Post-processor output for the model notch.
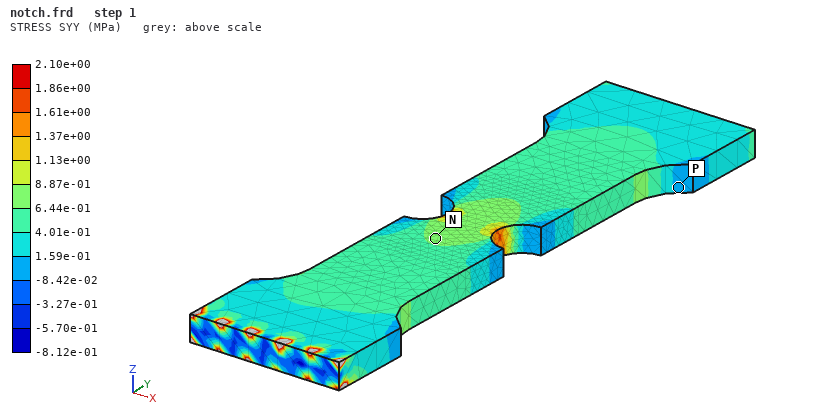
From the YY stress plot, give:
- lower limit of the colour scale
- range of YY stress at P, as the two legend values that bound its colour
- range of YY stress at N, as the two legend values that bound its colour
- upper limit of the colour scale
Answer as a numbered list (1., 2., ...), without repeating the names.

1. -8.12e-01 MPa
2. -8.42e-02 to 1.59e-01 MPa
3. 6.44e-01 to 8.87e-01 MPa
4. 2.10e+00 MPa
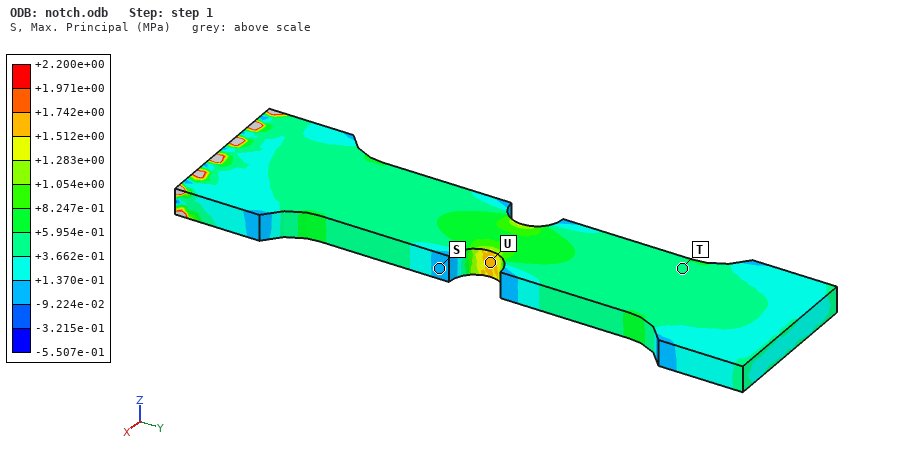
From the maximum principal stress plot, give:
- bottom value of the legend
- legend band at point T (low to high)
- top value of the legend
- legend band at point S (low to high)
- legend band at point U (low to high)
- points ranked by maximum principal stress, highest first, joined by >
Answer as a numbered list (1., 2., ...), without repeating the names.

1. -5.507e-01 MPa
2. +3.662e-01 to +5.954e-01 MPa
3. +2.200e+00 MPa
4. -9.224e-02 to +1.370e-01 MPa
5. +1.512e+00 to +1.742e+00 MPa
6. U > T > S
